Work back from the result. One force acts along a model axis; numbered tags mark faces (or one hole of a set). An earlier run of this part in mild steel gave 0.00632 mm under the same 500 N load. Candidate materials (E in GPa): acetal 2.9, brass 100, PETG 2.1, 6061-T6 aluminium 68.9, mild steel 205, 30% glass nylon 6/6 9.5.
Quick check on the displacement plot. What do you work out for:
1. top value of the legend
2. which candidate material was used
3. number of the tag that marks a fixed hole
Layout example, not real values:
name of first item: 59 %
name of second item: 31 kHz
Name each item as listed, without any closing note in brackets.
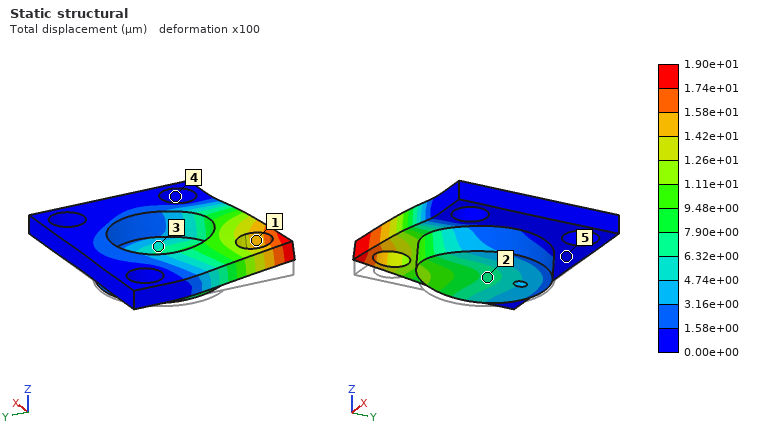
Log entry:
top value of the legend: 1.90e+01 µm
which candidate material was used: 6061-T6 aluminium
number of the tag that marks a fixed hole: 4
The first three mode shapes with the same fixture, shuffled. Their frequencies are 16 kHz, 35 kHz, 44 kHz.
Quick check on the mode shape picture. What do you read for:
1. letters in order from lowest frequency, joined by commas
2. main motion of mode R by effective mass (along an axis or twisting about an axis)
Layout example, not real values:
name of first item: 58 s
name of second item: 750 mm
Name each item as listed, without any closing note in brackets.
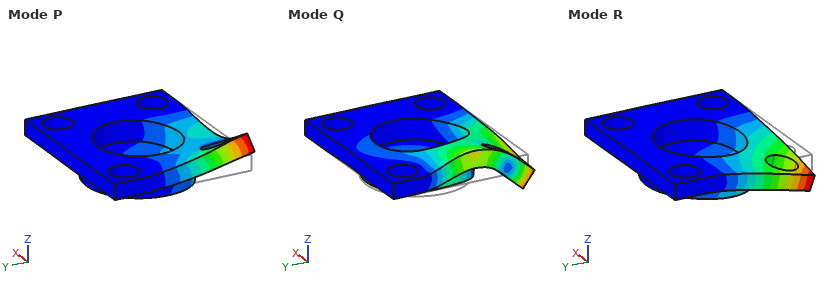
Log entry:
letters in order from lowest frequency, joined by commas: R, P, Q
main motion of mode R by effective mass: along Z
